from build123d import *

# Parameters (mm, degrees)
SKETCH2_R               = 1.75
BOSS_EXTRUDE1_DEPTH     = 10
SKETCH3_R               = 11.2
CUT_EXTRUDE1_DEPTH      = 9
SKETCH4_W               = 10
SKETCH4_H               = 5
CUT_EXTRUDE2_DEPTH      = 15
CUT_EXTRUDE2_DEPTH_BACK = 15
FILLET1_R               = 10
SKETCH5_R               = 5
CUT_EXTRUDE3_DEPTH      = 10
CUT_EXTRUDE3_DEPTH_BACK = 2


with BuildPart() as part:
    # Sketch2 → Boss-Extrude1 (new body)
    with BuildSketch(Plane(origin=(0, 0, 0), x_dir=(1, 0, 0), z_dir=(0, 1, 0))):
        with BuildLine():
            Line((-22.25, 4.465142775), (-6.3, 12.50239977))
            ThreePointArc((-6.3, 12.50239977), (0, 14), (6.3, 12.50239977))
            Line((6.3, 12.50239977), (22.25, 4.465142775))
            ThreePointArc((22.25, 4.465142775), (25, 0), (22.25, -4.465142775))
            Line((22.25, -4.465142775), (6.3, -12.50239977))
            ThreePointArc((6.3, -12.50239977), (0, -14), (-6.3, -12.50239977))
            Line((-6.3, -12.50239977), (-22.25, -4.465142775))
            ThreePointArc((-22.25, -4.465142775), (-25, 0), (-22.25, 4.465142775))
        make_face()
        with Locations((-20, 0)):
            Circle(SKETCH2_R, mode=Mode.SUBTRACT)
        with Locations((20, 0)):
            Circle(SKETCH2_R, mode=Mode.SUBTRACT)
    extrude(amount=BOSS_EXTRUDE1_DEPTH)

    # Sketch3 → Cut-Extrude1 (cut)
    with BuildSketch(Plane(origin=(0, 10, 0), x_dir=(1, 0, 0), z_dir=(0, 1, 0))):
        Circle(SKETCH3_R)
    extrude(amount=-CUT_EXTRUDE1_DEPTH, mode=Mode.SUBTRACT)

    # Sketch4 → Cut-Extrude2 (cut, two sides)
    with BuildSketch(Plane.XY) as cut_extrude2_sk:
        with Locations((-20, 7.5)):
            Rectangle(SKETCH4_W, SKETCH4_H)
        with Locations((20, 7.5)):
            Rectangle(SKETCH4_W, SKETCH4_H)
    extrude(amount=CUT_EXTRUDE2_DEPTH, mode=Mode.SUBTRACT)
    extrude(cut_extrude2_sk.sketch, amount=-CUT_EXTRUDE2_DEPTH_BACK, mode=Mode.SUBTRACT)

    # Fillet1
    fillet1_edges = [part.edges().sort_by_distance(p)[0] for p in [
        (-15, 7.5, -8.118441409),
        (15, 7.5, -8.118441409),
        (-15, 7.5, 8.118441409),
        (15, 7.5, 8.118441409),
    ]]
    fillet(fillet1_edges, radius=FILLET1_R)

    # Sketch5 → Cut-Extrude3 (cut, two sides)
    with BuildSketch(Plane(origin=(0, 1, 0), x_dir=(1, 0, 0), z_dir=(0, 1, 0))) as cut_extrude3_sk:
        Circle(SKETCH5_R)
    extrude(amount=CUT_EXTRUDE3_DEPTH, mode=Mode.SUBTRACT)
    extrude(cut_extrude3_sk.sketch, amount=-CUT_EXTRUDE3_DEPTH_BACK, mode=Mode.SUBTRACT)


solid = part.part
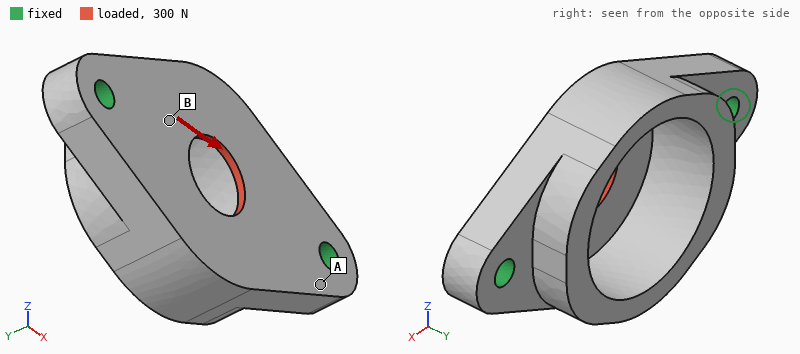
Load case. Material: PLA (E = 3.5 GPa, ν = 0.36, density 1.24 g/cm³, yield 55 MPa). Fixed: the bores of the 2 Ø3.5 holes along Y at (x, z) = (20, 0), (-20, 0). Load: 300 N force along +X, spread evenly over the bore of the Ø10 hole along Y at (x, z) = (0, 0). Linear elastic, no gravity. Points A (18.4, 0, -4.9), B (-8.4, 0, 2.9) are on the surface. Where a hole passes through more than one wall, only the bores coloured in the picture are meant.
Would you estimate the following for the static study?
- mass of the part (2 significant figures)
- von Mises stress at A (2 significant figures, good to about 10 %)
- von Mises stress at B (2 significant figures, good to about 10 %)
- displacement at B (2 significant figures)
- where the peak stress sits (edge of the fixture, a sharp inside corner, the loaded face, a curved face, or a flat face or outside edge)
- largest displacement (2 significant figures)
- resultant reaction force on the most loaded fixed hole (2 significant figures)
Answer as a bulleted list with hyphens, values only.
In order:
- 5.2 g
- 2.2 MPa
- 9.3 MPa
- 22 µm
- the loaded face
- 37 µm
- 150 N
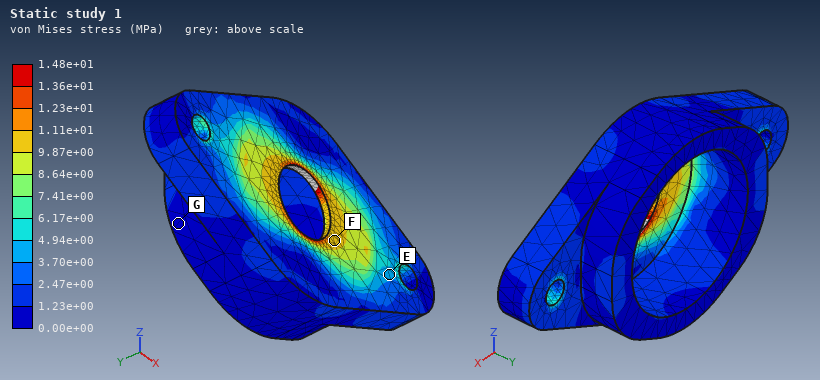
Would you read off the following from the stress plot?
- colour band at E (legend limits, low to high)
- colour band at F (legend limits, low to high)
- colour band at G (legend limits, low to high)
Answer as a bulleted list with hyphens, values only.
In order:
- 3.70e+00 to 4.94e+00 MPa
- 9.87e+00 to 1.11e+01 MPa
- 0.00e+00 to 1.23e+00 MPa
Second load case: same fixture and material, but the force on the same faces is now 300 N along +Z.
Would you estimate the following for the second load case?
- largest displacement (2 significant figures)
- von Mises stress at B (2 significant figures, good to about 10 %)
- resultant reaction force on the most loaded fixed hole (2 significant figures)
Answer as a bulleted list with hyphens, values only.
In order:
- 83 µm
- 7.7 MPa
- 150 N
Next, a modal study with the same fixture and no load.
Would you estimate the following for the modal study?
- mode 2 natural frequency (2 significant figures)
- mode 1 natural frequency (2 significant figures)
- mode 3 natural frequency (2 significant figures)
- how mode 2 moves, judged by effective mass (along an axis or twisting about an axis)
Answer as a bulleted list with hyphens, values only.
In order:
- 4400 Hz
- 3600 Hz
- 7400 Hz
- along Y
